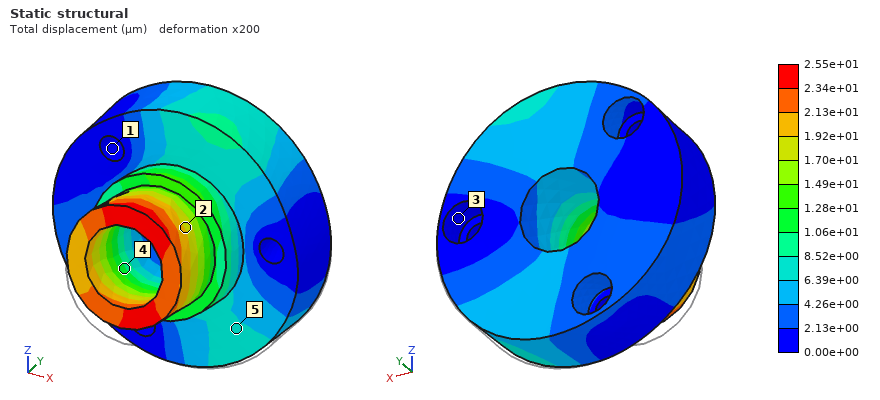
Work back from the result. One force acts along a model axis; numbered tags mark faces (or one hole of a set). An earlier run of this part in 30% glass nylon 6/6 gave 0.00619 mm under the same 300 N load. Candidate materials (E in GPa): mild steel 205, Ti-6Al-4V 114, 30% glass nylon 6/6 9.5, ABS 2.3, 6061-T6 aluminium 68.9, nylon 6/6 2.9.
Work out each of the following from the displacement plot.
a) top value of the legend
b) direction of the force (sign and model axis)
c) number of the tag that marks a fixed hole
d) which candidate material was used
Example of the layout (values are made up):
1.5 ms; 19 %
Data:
2.55e+01 µm; +Z; 1; ABS
